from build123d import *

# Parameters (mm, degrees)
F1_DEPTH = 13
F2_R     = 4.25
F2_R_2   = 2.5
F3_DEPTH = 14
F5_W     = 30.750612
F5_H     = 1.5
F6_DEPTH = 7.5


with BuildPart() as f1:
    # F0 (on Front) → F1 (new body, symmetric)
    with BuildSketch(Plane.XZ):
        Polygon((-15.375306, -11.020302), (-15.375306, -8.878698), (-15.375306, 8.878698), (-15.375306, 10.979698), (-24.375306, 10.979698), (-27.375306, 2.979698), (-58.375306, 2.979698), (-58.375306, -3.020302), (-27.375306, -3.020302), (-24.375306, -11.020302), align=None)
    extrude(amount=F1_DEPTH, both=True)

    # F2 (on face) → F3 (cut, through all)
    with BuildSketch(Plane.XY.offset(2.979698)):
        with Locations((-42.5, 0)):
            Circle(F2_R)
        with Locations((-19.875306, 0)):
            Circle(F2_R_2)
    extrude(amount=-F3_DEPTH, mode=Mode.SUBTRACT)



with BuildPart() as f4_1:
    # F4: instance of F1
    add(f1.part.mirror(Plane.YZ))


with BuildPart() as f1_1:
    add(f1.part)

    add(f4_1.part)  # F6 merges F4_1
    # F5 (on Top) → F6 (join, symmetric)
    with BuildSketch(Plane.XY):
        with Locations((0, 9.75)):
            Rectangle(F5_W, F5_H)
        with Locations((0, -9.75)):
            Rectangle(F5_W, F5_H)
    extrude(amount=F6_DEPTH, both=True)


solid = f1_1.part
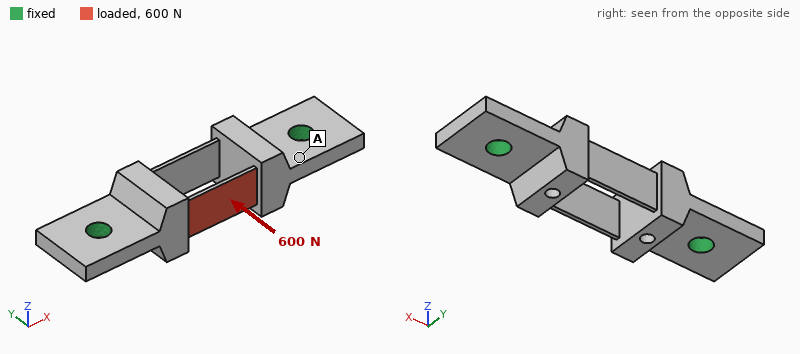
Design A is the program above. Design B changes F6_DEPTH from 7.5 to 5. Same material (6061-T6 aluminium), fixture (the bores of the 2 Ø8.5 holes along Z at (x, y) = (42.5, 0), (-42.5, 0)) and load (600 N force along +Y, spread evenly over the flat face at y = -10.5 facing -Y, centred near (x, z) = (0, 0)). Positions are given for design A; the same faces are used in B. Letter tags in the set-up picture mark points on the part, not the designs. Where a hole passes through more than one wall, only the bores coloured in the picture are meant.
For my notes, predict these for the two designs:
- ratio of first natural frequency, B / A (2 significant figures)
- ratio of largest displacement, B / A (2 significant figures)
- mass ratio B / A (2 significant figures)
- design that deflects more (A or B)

0.83
1.5
0.98
B
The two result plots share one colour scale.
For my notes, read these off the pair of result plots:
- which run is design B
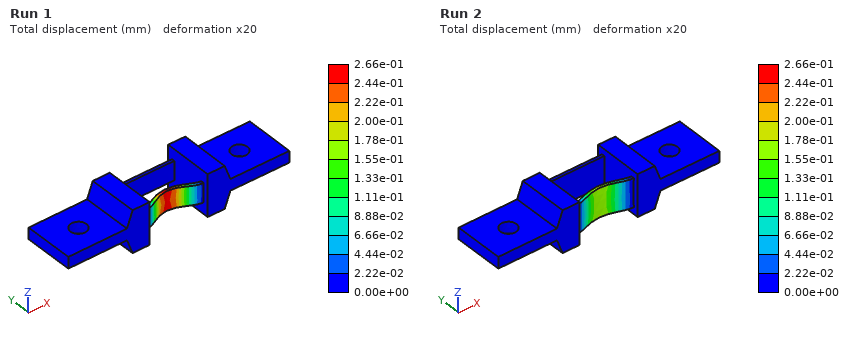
Run 1
